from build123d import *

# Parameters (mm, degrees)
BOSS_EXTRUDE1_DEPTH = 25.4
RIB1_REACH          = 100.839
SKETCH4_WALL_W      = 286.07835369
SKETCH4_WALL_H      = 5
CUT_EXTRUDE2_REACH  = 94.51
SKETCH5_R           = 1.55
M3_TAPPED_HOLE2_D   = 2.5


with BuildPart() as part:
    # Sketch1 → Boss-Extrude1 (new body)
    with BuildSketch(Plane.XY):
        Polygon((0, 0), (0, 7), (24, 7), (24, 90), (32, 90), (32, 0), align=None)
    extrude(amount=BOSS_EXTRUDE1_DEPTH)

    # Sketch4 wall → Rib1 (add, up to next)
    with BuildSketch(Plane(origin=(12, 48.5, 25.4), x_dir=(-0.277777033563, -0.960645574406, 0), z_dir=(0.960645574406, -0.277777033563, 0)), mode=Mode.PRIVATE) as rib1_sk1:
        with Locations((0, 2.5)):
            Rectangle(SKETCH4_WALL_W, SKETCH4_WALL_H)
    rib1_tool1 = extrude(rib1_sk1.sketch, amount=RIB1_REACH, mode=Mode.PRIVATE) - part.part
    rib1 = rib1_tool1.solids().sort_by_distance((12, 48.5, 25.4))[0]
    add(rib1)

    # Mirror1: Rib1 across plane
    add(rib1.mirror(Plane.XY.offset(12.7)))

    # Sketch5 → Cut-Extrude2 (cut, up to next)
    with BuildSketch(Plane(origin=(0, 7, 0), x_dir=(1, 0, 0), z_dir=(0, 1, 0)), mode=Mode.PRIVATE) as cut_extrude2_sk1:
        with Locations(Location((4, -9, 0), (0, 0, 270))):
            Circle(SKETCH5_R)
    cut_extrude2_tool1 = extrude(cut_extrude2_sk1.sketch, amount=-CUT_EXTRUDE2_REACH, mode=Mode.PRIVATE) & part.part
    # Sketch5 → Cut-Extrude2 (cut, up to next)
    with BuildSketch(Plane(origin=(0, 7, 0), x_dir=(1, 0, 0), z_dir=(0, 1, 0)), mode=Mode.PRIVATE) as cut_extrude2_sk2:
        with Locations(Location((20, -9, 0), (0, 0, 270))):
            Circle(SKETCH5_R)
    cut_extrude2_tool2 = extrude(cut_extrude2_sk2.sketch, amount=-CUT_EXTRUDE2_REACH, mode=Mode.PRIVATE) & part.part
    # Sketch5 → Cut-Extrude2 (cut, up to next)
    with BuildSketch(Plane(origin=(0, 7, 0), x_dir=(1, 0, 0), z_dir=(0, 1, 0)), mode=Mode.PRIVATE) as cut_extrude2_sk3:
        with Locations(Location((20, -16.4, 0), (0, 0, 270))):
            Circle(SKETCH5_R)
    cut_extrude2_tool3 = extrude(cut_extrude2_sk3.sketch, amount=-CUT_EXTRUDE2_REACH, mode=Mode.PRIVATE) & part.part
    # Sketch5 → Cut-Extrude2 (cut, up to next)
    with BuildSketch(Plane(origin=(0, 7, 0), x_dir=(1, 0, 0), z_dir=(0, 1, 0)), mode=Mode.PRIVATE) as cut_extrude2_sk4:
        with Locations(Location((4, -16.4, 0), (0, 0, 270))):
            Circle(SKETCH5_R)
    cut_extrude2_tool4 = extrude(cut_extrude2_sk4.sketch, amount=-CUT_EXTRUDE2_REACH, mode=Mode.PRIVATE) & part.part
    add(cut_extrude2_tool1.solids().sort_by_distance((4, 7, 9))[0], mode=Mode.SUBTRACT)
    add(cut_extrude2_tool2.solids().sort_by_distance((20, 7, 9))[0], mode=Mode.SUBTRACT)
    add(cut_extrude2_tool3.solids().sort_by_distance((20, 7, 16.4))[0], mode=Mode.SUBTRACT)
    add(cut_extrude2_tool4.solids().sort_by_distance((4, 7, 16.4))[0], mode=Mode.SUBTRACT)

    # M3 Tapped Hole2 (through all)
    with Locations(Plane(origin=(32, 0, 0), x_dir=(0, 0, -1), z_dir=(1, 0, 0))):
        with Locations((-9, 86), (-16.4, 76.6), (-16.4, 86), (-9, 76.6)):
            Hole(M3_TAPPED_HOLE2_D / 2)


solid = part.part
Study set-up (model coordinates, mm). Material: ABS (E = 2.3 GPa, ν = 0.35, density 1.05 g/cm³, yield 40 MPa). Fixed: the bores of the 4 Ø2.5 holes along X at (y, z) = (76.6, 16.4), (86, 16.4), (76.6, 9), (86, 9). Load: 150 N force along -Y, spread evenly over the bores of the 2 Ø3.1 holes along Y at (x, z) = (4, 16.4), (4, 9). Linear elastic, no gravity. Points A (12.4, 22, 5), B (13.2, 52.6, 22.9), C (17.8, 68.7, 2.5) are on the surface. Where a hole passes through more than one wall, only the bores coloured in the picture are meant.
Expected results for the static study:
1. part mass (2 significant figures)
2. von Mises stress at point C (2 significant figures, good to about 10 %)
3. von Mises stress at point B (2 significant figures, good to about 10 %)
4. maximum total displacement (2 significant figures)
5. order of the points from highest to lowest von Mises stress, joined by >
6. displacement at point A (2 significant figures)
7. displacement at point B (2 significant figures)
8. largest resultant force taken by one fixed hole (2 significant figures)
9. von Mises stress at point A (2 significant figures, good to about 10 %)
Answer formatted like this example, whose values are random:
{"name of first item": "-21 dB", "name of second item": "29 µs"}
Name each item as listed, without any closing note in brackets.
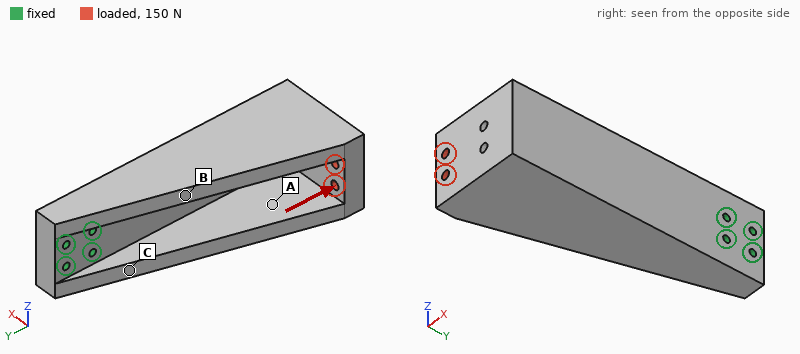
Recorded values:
{"part mass": "34 g", "von Mises stress at point C": "7.7 MPa", "von Mises stress at point B": "4.7 MPa", "maximum total displacement": "1.1 mm", "order of the points from highest to lowest von Mises stress, joined by >": "C > B > A", "displacement at point A": "0.67 mm", "displacement at point B": "0.27 mm", "largest resultant force taken by one fixed hole": "93 N", "von Mises stress at point A": "1.5 MPa"}
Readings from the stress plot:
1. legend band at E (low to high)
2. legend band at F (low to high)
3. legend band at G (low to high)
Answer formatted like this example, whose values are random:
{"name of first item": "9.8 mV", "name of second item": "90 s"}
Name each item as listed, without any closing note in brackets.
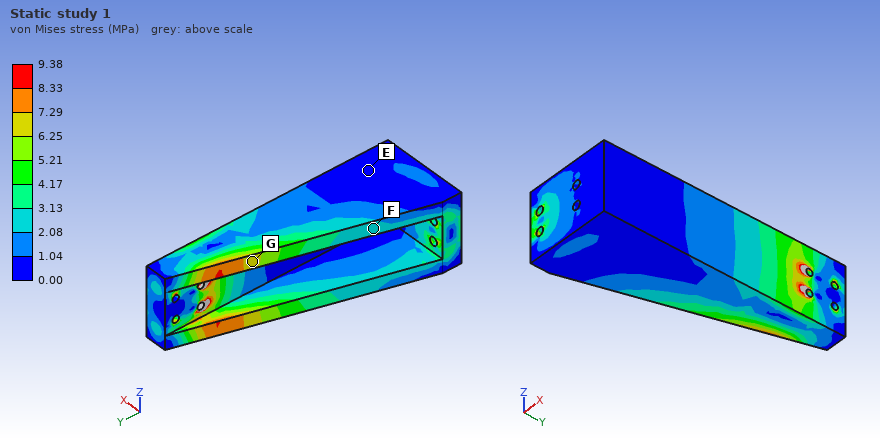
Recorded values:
{"legend band at E": "0.00 to 1.04 MPa", "legend band at F": "2.08 to 3.13 MPa", "legend band at G": "6.25 to 7.29 MPa"}
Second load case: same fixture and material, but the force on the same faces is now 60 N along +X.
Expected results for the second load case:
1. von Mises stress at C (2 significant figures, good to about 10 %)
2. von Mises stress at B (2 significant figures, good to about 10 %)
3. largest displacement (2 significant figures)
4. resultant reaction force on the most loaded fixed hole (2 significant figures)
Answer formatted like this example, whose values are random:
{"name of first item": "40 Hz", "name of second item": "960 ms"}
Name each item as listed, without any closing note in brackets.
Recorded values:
{"von Mises stress at C": "8.1 MPa", "von Mises stress at B": "3.8 MPa", "largest displacement": "1.2 mm", "resultant reaction force on the most loaded fixed hole": "120 N"}
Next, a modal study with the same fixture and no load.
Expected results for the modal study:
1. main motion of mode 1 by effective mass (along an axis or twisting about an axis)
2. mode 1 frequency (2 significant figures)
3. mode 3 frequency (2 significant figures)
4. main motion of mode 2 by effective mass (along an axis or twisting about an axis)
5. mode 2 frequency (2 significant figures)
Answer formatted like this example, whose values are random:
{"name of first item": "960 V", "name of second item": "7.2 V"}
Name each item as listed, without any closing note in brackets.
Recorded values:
{"main motion of mode 1 by effective mass": "along X", "mode 1 frequency": "330 Hz", "mode 3 frequency": "970 Hz", "main motion of mode 2 by effective mass": "along Z", "mode 2 frequency": "520 Hz"}
